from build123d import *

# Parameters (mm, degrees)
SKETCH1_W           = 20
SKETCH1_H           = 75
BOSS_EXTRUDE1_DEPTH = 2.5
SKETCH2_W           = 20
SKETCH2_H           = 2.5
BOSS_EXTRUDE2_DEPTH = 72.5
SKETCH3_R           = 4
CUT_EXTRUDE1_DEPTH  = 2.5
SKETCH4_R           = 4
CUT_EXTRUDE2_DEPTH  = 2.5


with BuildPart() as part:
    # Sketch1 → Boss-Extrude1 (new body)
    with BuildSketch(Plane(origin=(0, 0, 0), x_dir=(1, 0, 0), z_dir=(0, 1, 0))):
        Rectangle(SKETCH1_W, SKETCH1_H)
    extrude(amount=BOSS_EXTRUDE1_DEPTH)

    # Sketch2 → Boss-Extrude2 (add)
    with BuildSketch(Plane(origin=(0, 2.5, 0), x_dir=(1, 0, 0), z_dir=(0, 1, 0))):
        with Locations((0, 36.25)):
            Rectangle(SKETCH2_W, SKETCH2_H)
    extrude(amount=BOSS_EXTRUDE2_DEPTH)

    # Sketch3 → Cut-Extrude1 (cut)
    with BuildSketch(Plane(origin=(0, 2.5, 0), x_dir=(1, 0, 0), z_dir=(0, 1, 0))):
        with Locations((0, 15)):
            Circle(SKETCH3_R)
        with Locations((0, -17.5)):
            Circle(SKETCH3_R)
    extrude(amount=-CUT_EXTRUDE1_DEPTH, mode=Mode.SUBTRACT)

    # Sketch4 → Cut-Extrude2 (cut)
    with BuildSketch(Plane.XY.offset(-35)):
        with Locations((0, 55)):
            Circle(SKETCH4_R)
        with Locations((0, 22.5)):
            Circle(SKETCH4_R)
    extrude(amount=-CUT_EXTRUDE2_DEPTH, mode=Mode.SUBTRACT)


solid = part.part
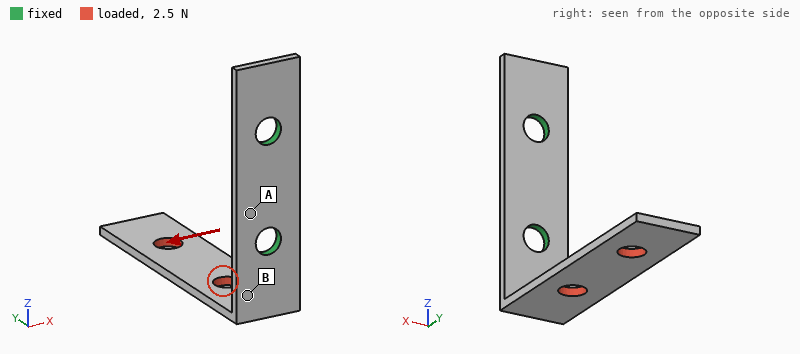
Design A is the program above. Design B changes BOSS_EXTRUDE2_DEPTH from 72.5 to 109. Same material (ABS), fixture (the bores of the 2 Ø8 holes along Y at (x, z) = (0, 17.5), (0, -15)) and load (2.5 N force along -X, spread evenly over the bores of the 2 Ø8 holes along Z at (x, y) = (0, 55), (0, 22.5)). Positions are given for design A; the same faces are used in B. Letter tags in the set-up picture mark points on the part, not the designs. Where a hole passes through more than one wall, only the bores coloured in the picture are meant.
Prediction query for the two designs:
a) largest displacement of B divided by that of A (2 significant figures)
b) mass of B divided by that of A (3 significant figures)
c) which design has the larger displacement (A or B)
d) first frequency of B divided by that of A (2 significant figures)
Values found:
1.5
1.27
B
0.47
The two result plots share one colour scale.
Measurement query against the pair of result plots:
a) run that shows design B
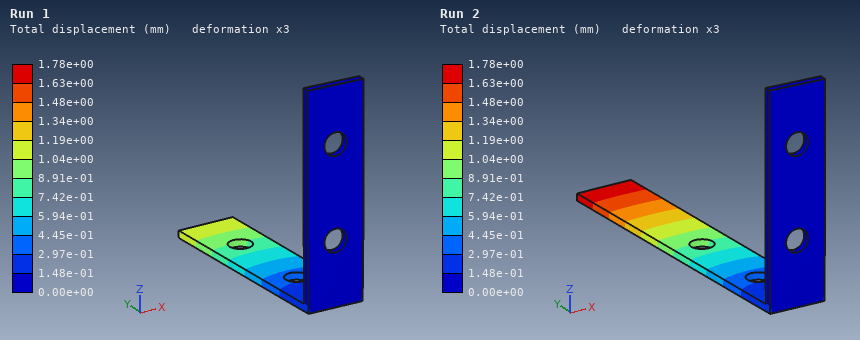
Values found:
Run 2
